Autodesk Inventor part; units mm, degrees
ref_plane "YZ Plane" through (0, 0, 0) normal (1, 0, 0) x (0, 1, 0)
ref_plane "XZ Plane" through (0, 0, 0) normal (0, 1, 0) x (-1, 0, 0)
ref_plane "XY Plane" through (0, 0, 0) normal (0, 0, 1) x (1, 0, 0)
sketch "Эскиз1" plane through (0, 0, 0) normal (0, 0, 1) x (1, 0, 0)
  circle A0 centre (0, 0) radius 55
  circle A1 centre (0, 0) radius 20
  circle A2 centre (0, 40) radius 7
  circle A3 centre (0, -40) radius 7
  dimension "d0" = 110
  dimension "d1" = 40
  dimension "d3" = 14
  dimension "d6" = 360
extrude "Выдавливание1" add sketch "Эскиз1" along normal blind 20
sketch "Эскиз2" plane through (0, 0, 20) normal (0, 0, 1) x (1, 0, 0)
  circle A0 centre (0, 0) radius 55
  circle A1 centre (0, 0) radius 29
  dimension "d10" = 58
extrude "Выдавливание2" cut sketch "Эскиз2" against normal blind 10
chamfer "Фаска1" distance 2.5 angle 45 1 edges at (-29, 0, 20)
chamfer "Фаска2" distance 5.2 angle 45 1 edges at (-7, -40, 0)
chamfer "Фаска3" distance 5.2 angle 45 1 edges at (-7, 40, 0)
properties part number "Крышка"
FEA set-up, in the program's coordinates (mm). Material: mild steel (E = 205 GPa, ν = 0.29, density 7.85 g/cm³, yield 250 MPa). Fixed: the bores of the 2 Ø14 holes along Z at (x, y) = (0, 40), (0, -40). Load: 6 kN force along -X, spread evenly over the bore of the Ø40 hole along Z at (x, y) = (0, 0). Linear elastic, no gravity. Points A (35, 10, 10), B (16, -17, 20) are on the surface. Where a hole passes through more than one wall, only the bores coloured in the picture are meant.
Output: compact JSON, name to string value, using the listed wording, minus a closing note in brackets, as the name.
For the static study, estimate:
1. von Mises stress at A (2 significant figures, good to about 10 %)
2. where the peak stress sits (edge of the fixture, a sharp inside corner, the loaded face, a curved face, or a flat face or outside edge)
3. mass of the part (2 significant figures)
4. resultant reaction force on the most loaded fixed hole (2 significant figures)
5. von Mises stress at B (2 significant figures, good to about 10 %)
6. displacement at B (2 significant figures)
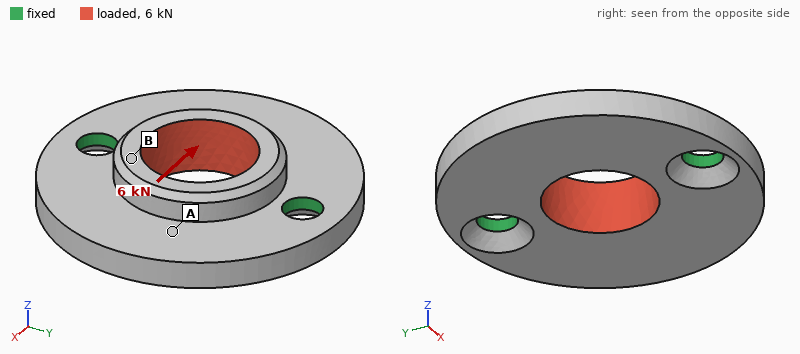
{"von Mises stress at A": "3.2 MPa", "where the peak stress sits": "edge of the fixture", "mass of the part": "720 g", "resultant reaction force on the most loaded fixed hole": "3.0 kN", "von Mises stress at B": "5.5 MPa", "displacement at B": "4.0 µm"}
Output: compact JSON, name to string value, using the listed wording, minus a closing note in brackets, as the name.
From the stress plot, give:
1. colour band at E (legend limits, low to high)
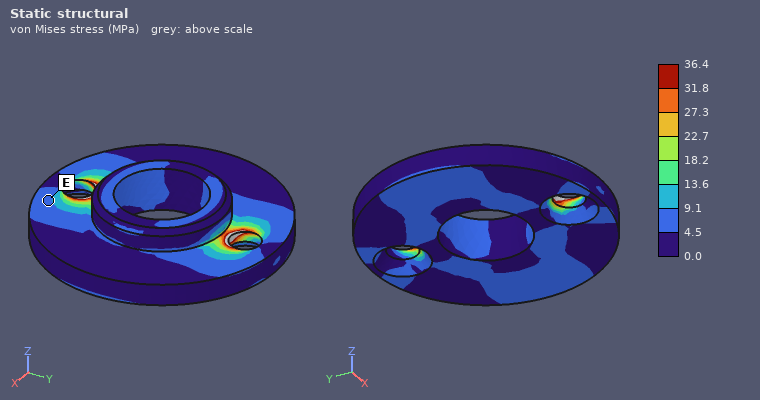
{"colour band at E": "4.5 to 9.1 MPa"}
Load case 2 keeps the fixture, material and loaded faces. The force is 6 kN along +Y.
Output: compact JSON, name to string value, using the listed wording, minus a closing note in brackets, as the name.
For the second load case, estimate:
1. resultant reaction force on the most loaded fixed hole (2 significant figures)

{"resultant reaction force on the most loaded fixed hole": "3.0 kN"}
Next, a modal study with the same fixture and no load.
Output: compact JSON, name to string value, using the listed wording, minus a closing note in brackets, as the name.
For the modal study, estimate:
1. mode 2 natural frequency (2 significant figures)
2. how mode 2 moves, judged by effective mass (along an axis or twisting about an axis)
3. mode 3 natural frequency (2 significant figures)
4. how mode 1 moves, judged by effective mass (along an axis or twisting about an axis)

{"mode 2 natural frequency": "3400 Hz", "how mode 2 moves, judged by effective mass": "along Z", "mode 3 natural frequency": "6600 Hz", "how mode 1 moves, judged by effective mass": "twisting about Y"}
